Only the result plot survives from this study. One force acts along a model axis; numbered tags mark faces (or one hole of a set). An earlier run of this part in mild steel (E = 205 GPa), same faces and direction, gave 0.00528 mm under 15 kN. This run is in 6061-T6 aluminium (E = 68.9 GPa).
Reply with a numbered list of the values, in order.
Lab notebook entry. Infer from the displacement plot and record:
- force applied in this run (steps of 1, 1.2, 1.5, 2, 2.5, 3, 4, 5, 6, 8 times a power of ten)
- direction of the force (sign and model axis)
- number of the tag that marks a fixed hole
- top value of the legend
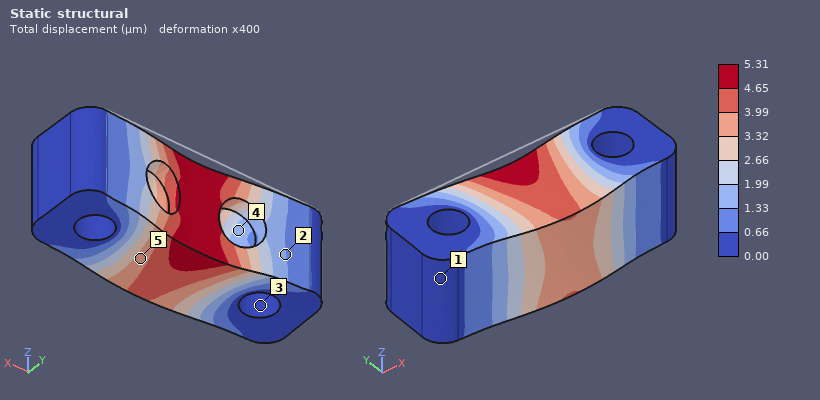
1. 5 kN
2. -Y
3. 3
4. 5.31 µm
